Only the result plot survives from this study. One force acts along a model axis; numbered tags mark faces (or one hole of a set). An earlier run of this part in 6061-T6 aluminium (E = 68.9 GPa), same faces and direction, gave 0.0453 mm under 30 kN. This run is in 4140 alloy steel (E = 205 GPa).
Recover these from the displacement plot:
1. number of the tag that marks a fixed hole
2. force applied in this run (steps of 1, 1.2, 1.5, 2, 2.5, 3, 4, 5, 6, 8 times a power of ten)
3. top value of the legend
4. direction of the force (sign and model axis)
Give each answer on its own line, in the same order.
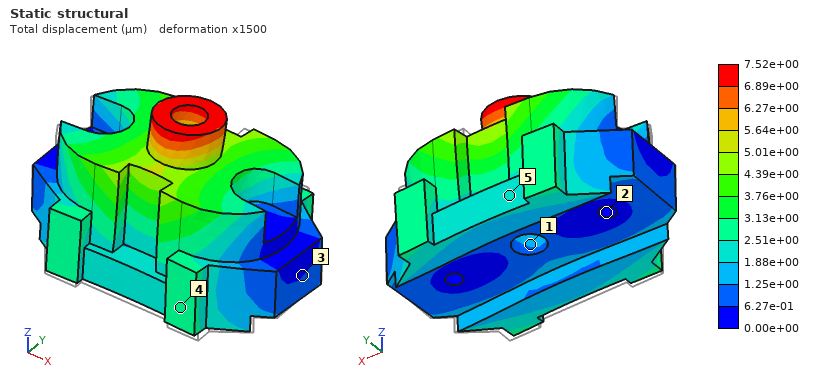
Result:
2
15 kN
7.52e+00 µm
+Y
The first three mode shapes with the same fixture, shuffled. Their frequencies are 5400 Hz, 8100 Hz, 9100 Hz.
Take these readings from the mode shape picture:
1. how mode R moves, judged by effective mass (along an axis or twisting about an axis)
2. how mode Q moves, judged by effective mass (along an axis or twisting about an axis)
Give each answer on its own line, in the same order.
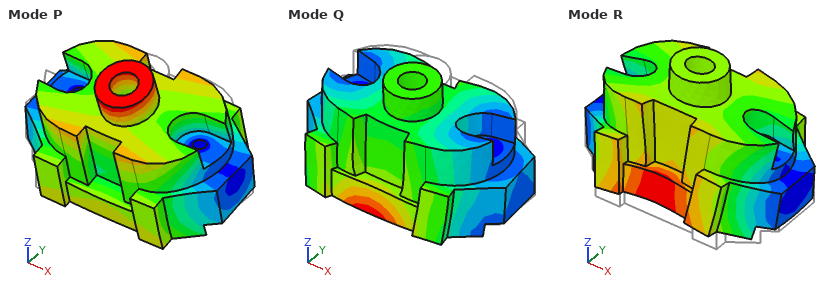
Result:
along Z
along Y
